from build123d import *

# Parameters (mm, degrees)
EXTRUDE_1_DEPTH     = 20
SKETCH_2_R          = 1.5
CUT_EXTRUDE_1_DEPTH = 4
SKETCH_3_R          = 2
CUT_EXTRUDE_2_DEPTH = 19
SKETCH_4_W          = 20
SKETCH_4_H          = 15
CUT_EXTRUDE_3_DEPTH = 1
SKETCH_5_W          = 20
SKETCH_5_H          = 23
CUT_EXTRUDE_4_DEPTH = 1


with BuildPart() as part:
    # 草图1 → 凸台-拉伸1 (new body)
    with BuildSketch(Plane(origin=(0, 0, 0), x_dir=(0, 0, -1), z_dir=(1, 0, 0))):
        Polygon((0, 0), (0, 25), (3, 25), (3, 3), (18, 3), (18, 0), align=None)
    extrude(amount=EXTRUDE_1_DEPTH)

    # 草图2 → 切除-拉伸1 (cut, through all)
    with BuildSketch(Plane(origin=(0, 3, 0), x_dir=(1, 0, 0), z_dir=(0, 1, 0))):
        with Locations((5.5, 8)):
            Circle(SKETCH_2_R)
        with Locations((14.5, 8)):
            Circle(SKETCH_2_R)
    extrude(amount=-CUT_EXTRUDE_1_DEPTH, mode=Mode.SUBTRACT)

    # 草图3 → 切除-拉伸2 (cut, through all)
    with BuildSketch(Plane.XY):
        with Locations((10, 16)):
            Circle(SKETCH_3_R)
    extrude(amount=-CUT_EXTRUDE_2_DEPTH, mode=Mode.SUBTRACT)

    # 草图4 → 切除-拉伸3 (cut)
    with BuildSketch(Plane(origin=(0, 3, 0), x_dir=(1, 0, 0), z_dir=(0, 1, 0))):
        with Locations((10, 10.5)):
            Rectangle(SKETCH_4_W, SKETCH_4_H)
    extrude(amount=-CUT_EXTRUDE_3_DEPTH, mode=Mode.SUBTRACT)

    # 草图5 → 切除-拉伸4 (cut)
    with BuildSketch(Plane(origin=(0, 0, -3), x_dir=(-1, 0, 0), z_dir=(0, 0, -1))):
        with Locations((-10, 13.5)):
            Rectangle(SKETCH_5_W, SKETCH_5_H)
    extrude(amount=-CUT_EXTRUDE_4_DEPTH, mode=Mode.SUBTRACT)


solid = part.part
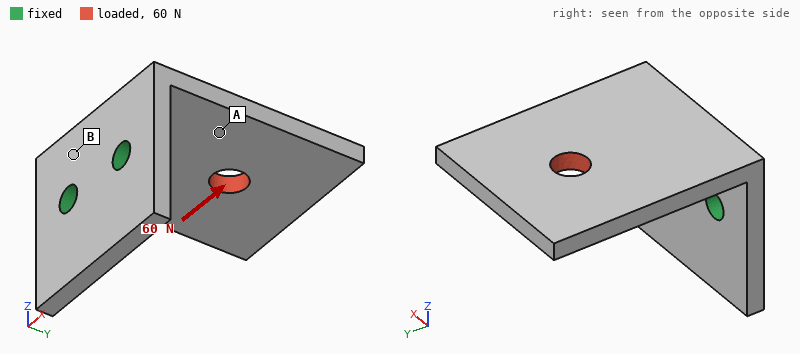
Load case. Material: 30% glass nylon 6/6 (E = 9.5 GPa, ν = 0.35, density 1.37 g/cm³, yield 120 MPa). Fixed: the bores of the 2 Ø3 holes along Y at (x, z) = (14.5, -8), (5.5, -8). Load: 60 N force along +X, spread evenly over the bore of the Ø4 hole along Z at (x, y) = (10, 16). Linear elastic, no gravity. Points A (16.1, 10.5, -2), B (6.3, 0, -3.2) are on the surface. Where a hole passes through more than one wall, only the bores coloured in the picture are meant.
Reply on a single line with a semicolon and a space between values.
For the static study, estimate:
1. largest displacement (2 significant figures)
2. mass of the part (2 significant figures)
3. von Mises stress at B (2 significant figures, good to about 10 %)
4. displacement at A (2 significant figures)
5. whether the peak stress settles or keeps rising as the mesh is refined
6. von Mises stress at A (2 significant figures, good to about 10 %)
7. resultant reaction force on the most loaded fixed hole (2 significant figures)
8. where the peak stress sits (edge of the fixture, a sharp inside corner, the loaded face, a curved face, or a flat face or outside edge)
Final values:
0.28 mm; 2.2 g; 18 MPa; 0.13 mm; keeps rising; 6.7 MPa; 86 N; edge of the fixture
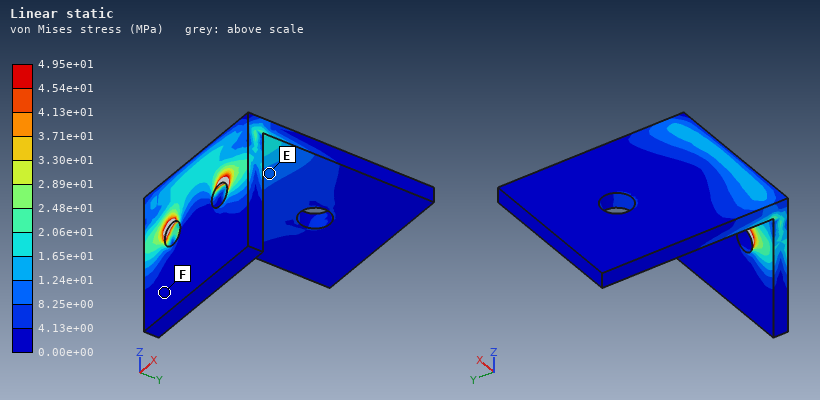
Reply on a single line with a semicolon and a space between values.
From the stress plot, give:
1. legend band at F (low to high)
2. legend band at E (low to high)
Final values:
0.00e+00 to 4.13e+00 MPa; 8.25e+00 to 1.24e+01 MPa
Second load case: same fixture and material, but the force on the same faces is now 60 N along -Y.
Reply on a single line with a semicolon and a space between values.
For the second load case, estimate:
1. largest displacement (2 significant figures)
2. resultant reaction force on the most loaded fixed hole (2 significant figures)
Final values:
0.22 mm; 30 N
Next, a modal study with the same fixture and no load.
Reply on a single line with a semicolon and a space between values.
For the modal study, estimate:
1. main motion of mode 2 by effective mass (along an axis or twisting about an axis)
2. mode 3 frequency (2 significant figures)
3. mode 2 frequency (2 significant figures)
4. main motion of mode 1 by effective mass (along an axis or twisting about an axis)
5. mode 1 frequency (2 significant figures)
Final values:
along X; 3900 Hz; 2600 Hz; along Z; 1100 Hz
